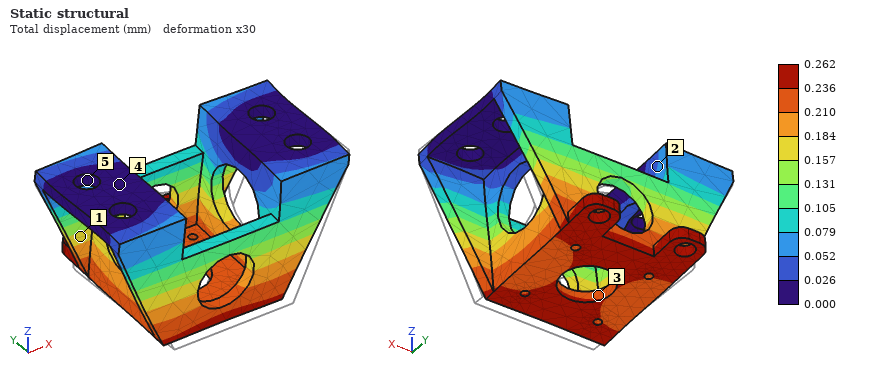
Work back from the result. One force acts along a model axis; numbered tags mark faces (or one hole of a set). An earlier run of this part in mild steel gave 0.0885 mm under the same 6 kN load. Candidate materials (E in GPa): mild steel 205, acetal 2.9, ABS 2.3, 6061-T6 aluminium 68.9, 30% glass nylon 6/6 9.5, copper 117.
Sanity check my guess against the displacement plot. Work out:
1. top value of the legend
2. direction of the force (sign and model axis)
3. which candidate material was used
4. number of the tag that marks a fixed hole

0.262 mm
+Y
6061-T6 aluminium
5
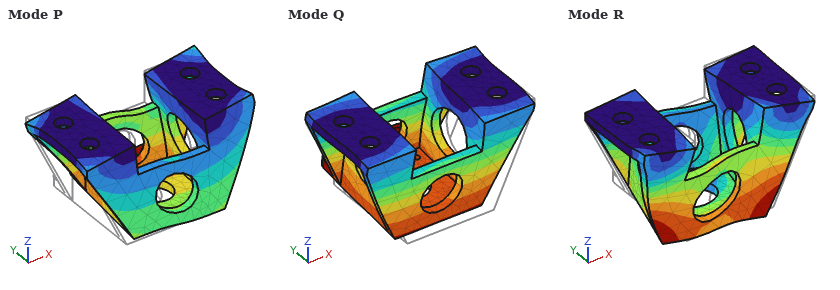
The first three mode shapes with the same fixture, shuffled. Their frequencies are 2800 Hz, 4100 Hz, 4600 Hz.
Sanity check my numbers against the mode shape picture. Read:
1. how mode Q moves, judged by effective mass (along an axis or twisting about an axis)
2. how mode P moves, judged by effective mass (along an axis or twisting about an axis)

along Y
along X
